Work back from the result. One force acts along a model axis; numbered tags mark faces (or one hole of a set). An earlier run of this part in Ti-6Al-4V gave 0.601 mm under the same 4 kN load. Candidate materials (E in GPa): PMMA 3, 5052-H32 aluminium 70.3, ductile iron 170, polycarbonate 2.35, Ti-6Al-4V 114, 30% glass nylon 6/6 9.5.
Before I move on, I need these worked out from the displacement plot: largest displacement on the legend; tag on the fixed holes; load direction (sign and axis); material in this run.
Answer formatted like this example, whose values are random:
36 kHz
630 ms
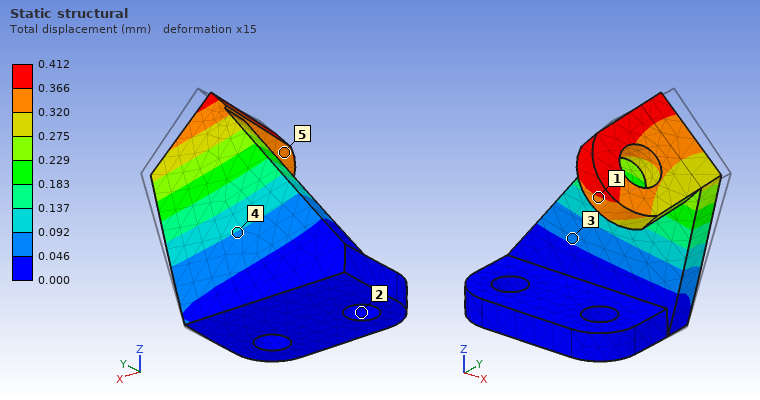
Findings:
0.412 mm
2
-Y
ductile iron
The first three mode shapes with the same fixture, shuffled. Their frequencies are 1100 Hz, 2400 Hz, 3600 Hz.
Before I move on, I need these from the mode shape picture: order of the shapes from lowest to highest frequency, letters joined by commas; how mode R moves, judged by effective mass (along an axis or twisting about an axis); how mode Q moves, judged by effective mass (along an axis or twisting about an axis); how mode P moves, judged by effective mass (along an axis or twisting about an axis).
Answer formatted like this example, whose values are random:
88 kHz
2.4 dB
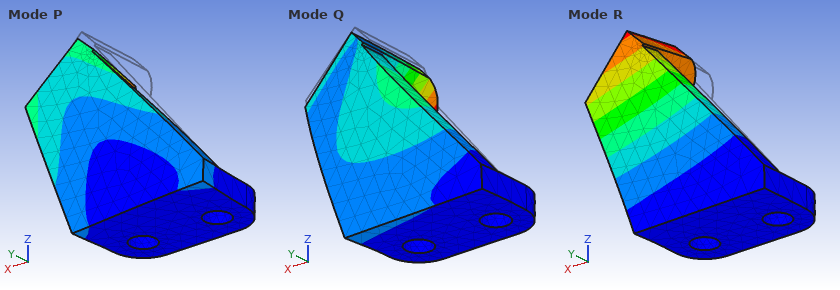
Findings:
R, P, Q
along Y
along Z
along X
